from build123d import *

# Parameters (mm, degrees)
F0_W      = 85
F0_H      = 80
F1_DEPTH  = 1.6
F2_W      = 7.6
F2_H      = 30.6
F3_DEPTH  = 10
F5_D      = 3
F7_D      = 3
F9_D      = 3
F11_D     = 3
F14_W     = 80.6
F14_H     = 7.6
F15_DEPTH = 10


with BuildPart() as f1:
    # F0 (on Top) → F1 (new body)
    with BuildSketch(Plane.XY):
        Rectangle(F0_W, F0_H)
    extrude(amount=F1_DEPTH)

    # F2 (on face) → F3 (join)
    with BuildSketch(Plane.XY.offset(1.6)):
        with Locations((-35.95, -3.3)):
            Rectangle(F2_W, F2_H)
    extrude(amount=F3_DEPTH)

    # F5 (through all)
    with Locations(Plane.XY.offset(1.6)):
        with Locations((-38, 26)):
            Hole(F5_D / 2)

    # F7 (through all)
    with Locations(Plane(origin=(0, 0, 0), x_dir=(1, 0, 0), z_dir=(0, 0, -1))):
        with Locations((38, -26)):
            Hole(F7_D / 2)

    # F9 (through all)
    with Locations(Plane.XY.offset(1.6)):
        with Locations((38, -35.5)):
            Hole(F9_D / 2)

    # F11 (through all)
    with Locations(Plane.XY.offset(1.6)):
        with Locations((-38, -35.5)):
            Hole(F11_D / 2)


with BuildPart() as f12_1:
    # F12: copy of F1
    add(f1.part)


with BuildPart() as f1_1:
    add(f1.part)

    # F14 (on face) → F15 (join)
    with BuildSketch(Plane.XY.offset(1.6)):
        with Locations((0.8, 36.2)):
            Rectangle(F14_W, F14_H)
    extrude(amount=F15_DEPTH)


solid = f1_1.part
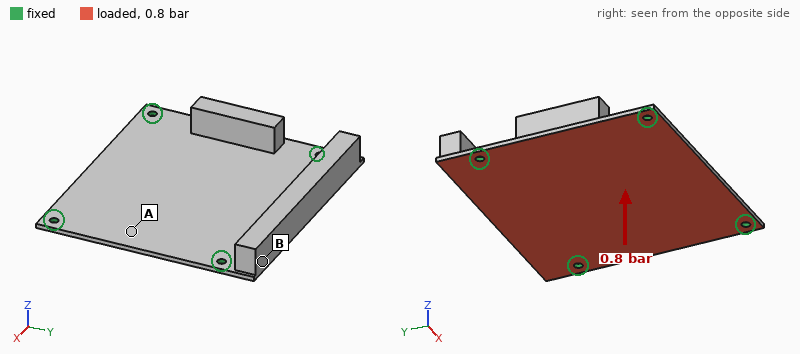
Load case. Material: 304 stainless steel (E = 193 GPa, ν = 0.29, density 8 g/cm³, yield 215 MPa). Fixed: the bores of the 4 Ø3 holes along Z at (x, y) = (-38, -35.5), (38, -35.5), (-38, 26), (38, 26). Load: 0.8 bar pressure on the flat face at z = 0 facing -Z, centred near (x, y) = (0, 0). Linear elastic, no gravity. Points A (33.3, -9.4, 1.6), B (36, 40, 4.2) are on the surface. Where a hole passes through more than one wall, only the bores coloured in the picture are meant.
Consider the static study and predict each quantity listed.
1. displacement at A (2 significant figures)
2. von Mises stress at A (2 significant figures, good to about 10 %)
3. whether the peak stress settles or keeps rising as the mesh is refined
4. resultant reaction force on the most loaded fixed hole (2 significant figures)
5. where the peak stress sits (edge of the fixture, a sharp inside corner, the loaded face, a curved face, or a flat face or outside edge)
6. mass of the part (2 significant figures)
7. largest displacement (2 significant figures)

0.076 mm
39 MPa
keeps rising
190 N
edge of the fixture
150 g
0.15 mm
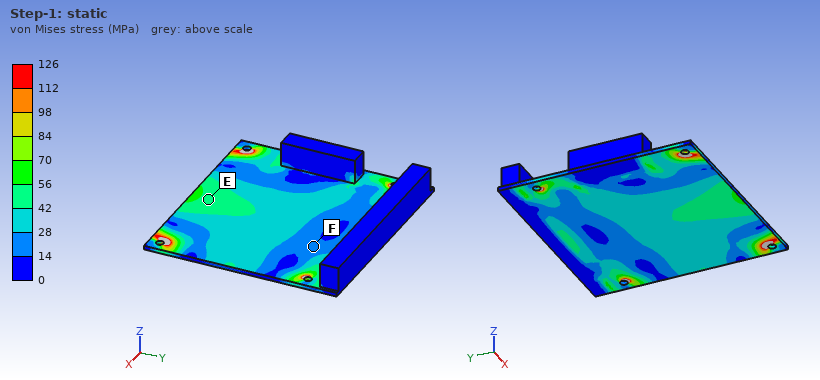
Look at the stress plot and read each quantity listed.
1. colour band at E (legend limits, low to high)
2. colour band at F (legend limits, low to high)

42 to 56 MPa
14 to 28 MPa
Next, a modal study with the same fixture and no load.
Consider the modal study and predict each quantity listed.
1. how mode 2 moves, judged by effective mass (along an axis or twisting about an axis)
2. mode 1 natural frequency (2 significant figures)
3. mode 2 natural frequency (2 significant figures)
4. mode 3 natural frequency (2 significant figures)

along Z
1200 Hz
1600 Hz
2200 Hz
